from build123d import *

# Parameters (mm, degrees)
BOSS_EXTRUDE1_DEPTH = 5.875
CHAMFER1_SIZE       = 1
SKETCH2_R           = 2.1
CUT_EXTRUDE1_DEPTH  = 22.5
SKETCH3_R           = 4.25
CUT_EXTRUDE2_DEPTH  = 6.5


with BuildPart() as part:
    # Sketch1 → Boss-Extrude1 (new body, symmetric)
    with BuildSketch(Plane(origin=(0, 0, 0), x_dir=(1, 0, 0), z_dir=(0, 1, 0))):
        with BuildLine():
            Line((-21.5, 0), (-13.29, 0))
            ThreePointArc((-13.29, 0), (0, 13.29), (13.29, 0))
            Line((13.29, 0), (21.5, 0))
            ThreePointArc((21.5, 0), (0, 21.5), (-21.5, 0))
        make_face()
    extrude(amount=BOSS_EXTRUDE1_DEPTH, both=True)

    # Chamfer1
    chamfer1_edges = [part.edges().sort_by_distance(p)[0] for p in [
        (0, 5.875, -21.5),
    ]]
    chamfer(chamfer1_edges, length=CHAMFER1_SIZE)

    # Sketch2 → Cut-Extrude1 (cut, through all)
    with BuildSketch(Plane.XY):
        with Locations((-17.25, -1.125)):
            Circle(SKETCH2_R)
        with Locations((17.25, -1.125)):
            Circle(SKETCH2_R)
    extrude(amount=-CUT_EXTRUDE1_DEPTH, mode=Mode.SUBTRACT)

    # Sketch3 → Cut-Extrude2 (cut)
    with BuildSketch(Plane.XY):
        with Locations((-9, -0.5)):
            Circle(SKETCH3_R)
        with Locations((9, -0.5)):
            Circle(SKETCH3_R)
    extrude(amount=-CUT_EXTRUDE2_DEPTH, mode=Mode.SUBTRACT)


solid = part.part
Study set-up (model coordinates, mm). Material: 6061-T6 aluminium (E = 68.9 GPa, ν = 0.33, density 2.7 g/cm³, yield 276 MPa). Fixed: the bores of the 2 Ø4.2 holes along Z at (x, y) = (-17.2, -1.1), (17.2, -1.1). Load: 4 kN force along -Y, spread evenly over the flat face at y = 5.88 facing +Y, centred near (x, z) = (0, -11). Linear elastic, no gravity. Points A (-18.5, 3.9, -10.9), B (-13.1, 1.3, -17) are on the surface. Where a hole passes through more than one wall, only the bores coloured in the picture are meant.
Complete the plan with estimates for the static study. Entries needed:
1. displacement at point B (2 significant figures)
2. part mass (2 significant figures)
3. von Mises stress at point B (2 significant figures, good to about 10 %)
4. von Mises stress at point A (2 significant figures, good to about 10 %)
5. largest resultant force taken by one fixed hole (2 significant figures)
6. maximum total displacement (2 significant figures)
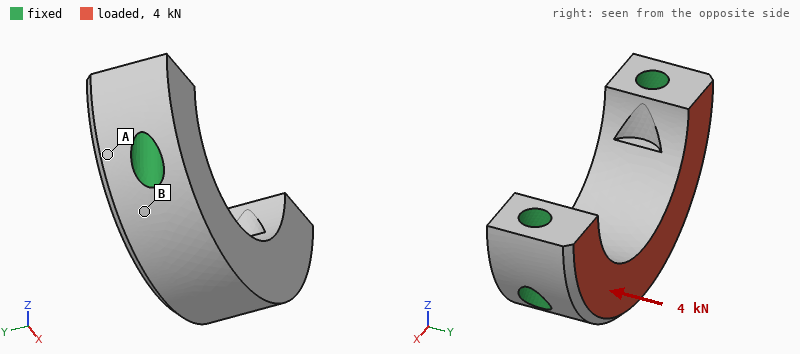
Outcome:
6.4 µm
13 g
35 MPa
16 MPa
2.0 kN
18 µm
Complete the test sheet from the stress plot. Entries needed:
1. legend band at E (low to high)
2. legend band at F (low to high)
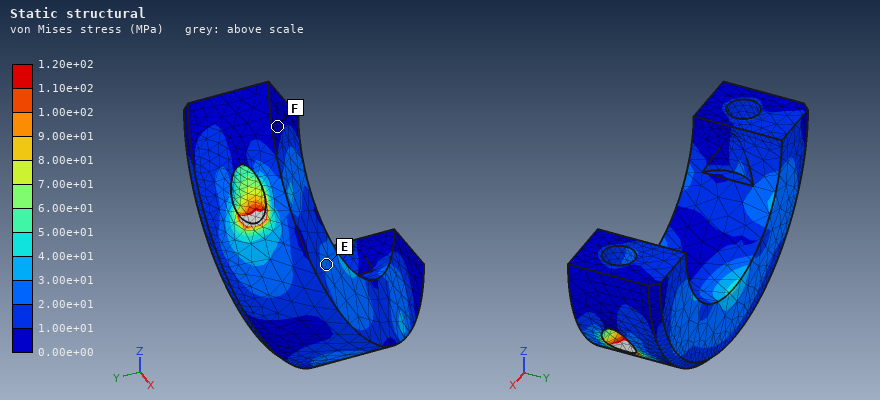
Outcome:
2.00e+01 to 3.00e+01 MPa
0.00e+00 to 1.00e+01 MPa
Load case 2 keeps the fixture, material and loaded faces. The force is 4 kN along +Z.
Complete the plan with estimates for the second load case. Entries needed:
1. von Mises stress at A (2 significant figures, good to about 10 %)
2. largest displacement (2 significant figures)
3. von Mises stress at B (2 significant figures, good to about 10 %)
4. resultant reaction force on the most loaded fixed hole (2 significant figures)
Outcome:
22 MPa
23 µm
32 MPa
2.1 kN
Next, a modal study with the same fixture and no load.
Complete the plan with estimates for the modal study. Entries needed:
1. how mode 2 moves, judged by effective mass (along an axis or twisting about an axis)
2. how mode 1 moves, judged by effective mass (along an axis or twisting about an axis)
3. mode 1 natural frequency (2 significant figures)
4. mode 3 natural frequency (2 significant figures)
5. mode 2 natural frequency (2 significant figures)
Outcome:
along Z
along Y
24 kHz
50 kHz
39 kHz
